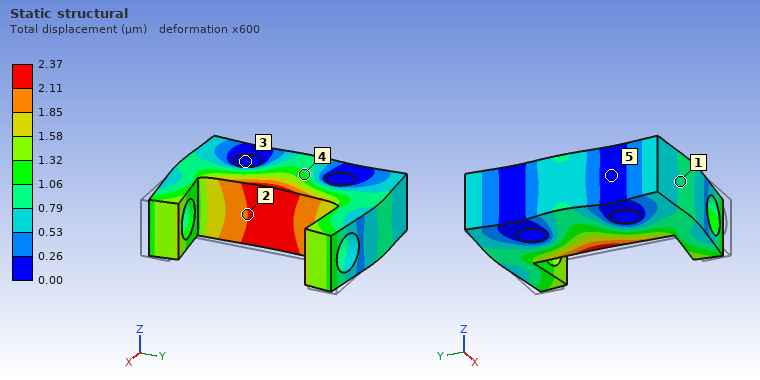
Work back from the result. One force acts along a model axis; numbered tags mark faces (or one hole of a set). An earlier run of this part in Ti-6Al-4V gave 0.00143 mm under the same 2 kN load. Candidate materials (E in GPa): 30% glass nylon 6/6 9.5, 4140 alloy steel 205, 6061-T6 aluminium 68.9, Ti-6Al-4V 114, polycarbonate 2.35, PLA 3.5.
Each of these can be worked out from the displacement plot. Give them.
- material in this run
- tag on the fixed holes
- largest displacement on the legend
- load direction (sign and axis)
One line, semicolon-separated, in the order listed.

6061-T6 aluminium; 3; 2.37 µm; -X
